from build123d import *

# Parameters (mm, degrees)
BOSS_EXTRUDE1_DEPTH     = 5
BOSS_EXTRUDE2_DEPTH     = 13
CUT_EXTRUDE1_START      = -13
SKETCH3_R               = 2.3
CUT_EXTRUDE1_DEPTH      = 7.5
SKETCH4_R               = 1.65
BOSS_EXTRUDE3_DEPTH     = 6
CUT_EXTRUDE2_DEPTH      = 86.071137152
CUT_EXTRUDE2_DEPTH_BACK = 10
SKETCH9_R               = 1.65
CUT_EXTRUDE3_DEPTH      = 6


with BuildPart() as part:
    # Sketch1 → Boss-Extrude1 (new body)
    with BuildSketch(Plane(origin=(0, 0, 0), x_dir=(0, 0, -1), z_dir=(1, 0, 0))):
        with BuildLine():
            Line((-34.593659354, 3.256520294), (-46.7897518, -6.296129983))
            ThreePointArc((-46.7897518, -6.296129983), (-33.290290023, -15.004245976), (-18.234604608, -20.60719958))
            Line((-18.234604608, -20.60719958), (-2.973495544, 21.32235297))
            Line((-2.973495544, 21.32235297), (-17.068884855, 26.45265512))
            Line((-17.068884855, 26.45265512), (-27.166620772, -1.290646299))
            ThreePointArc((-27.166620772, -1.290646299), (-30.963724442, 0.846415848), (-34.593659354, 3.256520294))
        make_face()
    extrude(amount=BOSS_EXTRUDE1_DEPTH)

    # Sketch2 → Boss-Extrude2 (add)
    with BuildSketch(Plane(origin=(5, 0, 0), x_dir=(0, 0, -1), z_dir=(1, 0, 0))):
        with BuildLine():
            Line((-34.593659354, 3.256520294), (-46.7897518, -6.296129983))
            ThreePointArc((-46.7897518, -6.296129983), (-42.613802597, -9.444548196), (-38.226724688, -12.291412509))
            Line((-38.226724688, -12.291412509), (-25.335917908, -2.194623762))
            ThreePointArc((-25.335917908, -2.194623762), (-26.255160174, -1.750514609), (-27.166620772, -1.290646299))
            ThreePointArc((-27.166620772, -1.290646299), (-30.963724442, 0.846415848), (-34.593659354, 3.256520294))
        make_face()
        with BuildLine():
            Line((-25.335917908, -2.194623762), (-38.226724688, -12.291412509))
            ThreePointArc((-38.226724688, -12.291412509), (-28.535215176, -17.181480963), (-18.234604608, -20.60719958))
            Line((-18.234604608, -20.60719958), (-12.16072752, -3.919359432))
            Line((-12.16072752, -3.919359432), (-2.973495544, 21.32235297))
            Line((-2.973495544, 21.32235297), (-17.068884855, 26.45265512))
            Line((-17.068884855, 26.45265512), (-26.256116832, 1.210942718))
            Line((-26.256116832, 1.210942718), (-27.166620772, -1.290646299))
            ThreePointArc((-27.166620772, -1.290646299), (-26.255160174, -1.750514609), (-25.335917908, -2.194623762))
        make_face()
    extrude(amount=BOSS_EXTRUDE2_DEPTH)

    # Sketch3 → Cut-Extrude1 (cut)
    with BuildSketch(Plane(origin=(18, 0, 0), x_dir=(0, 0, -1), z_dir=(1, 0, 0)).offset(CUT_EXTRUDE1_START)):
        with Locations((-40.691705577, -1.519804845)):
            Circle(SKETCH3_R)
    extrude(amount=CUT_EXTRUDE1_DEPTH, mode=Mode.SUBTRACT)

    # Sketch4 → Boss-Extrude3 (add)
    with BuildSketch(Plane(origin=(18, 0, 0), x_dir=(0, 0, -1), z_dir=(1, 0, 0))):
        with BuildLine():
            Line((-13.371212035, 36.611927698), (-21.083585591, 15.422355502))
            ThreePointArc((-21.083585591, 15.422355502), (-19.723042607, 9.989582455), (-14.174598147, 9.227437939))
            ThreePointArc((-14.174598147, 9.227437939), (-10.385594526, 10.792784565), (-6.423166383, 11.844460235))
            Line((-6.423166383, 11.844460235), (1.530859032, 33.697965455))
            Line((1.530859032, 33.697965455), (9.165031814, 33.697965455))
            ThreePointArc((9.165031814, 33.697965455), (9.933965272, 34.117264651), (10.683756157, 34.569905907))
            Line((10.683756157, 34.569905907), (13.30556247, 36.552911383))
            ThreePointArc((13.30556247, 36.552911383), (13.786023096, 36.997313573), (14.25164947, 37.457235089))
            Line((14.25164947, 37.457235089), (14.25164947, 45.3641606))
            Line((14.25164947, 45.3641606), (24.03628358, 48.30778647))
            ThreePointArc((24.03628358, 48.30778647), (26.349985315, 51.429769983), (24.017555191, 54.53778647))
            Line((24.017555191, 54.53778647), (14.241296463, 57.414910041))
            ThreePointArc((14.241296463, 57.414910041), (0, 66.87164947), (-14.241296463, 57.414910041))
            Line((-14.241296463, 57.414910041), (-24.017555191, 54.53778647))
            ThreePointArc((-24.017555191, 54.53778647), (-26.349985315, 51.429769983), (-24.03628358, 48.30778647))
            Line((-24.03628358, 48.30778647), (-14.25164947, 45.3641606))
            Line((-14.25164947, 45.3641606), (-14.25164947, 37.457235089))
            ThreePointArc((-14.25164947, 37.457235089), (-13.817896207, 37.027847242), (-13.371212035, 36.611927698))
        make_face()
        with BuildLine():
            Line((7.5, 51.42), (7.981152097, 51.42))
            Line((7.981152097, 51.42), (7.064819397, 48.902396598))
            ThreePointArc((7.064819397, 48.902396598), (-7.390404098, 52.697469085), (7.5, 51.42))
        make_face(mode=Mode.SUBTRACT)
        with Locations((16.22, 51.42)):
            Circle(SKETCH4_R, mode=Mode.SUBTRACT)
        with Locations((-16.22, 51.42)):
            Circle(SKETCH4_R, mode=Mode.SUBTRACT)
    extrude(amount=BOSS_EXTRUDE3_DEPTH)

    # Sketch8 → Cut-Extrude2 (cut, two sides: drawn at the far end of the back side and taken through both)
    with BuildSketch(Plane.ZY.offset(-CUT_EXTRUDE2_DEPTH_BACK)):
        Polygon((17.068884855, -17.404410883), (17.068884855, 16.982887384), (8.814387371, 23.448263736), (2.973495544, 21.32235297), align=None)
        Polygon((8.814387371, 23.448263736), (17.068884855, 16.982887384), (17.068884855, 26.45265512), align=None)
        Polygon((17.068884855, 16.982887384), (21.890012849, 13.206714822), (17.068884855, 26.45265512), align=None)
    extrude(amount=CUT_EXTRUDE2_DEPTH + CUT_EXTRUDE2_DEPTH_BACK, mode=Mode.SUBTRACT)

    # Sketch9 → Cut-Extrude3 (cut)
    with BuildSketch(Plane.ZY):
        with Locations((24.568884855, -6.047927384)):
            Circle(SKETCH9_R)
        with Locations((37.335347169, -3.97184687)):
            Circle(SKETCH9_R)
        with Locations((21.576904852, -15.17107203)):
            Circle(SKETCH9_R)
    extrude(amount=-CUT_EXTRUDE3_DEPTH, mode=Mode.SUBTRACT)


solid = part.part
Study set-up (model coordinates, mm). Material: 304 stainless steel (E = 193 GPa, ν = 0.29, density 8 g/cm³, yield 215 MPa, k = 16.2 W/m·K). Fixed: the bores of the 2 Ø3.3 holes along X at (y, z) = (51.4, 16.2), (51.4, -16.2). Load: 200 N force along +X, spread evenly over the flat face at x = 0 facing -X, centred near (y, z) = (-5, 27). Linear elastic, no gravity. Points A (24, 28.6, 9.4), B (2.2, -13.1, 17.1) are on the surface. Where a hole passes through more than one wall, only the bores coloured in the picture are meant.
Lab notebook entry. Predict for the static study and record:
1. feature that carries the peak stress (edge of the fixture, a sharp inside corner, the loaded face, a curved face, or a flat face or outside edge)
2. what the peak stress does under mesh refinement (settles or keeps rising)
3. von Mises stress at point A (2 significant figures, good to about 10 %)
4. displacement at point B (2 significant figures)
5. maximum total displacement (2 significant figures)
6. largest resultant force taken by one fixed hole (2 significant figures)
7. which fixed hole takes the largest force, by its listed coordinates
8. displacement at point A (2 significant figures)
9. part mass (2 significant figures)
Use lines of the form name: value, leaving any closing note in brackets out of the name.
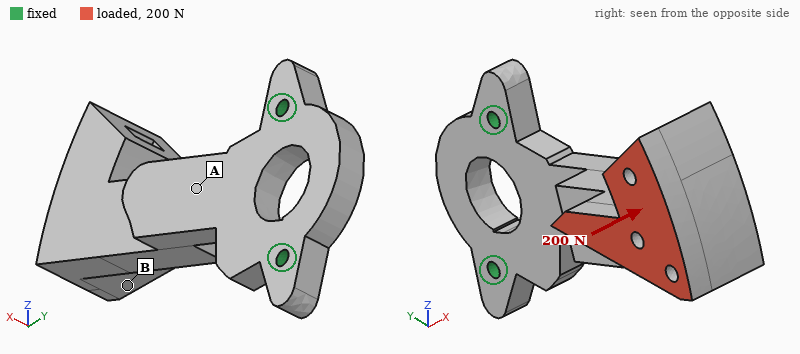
feature that carries the peak stress: edge of the fixture
what the peak stress does under mesh refinement: keeps rising
von Mises stress at point A: 81 MPa
displacement at point B: 0.29 mm
maximum total displacement: 0.34 mm
largest resultant force taken by one fixed hole: 290 N
which fixed hole takes the largest force, by its listed coordinates: (51.4, 16.2)
displacement at point A: 0.058 mm
part mass: 160 g
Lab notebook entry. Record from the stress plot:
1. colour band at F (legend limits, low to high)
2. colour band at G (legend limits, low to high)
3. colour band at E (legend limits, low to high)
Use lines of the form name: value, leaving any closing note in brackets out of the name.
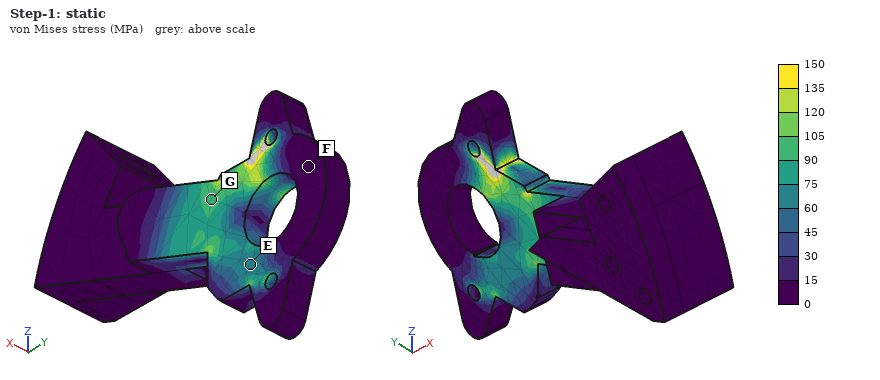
colour band at F: 0 to 15 MPa
colour band at G: 90 to 105 MPa
colour band at E: 60 to 75 MPa
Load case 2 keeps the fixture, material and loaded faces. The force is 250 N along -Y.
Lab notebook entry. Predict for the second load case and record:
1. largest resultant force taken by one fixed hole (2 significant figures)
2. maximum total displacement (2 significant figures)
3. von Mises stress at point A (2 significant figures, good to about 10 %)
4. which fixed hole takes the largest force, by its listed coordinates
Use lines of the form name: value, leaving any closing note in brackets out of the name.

largest resultant force taken by one fixed hole: 370 N
maximum total displacement: 0.19 mm
von Mises stress at point A: 50 MPa
which fixed hole takes the largest force, by its listed coordinates: (51.4, 16.2)
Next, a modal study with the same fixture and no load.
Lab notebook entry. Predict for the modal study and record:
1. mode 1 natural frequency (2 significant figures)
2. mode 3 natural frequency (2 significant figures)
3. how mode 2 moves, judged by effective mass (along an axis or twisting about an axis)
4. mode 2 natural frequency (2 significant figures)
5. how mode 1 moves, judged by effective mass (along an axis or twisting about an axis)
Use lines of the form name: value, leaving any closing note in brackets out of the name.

mode 1 natural frequency: 460 Hz
mode 3 natural frequency: 2900 Hz
how mode 2 moves, judged by effective mass: along Z
mode 2 natural frequency: 1200 Hz
how mode 1 moves, judged by effective mass: along X
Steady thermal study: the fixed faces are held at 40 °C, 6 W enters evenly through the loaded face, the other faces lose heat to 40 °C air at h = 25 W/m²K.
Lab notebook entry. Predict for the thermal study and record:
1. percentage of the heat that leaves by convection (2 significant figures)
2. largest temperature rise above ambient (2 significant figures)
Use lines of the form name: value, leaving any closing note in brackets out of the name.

percentage of the heat that leaves by convection: 82 %
largest temperature rise above ambient: 58 K
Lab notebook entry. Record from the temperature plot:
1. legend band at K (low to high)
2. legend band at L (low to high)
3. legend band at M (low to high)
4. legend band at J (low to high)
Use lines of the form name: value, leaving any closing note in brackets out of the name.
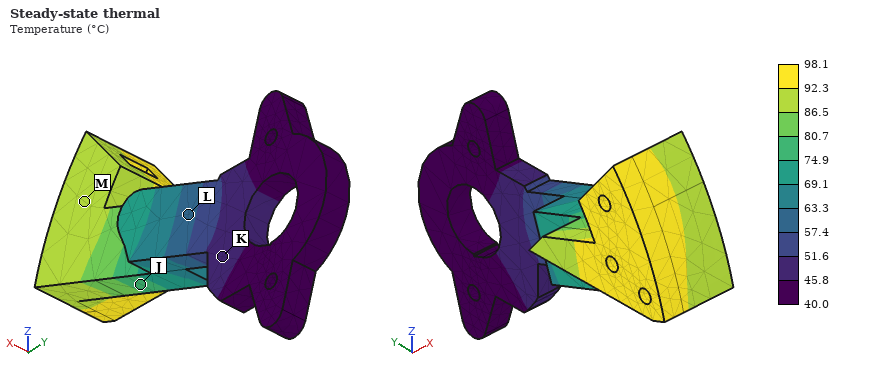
legend band at K: 45.8 to 51.6 °C
legend band at L: 57.4 to 63.3 °C
legend band at M: 86.5 to 92.3 °C
legend band at J: 74.9 to 80.7 °C
